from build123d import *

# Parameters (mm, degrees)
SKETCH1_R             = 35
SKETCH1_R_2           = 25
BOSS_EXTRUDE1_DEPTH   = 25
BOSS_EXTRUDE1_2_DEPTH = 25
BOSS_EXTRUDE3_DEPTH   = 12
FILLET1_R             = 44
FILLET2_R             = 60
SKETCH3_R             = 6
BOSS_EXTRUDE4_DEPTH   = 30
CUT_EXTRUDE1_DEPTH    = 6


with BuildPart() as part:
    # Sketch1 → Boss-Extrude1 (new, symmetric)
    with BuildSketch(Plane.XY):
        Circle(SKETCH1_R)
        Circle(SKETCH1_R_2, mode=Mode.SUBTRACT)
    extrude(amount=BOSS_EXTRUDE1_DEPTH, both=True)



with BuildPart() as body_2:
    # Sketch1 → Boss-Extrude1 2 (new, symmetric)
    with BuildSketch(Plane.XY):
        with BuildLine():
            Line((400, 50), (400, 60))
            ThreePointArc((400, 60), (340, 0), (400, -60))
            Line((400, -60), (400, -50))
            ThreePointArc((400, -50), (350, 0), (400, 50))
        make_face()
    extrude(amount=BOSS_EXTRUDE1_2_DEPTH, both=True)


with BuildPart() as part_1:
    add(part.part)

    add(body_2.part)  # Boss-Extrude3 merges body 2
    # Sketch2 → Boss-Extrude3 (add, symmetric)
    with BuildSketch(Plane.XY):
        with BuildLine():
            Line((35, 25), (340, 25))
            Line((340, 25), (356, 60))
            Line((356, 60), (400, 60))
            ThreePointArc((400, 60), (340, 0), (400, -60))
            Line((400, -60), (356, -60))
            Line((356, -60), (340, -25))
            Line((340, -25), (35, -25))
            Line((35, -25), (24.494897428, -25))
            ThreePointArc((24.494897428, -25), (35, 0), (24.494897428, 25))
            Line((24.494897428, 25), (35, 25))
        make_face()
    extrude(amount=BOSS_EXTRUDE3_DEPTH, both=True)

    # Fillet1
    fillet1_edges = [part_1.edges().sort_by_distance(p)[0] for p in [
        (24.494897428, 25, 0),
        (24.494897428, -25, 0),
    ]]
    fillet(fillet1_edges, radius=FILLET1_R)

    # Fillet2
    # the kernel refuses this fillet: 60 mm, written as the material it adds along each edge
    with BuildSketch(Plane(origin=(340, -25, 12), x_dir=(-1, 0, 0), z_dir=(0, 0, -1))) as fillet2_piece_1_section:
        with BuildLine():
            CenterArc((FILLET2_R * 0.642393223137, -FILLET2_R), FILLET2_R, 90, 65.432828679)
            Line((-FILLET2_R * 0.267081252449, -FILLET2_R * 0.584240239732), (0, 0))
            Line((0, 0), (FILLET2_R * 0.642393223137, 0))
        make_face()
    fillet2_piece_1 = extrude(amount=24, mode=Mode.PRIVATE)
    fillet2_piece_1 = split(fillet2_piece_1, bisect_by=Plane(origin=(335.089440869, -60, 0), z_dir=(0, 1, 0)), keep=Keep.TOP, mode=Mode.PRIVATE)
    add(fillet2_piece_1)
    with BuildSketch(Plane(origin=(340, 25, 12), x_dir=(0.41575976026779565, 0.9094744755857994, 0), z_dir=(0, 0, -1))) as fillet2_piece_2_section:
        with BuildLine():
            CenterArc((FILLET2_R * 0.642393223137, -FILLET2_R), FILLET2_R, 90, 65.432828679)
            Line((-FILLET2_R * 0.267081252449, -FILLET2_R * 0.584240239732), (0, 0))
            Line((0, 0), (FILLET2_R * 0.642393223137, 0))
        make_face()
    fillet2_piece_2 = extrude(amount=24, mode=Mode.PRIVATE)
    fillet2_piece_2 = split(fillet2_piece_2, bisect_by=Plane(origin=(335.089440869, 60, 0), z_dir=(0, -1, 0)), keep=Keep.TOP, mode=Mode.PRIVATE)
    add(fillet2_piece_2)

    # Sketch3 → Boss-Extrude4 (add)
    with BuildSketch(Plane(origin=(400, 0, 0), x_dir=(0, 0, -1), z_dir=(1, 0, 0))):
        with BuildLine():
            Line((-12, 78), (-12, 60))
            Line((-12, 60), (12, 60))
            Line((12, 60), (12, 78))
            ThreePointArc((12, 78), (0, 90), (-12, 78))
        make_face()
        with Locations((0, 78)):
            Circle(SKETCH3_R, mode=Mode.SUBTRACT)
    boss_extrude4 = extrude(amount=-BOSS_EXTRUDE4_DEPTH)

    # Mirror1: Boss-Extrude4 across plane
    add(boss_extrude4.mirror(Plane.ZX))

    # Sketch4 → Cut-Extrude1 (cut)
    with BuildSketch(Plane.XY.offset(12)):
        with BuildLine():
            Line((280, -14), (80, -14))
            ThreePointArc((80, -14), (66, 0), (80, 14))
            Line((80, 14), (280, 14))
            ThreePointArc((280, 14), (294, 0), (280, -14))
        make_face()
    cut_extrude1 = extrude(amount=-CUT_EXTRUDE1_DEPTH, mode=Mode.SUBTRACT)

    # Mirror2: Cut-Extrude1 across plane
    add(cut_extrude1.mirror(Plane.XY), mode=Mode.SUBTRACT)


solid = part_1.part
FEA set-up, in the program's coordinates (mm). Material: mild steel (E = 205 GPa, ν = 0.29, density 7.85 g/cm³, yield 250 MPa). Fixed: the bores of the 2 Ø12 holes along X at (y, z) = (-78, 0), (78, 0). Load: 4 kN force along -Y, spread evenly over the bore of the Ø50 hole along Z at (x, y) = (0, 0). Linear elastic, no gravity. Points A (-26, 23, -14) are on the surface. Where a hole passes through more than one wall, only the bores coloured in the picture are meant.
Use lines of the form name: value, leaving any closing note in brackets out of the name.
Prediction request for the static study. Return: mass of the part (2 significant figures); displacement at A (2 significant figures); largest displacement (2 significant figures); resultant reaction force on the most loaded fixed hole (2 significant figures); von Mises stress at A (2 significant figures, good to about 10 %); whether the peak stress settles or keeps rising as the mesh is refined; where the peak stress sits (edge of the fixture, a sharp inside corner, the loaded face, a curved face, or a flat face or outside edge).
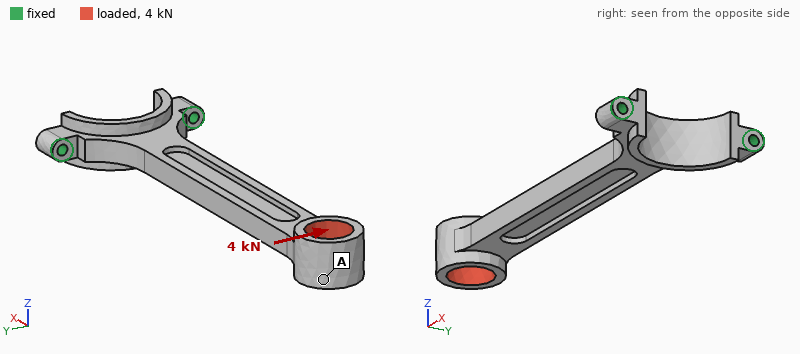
mass of the part: 4.3 kg
displacement at A: 1.5 mm
largest displacement: 1.5 mm
resultant reaction force on the most loaded fixed hole: 15 kN
von Mises stress at A: 12 MPa
whether the peak stress settles or keeps rising as the mesh is refined: keeps rising
where the peak stress sits: edge of the fixture
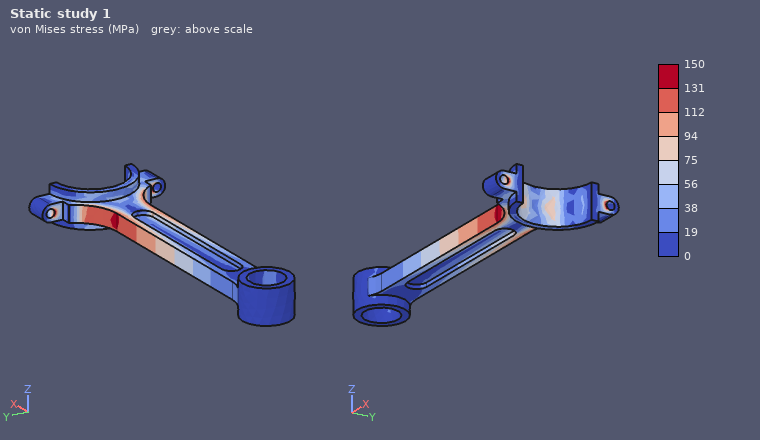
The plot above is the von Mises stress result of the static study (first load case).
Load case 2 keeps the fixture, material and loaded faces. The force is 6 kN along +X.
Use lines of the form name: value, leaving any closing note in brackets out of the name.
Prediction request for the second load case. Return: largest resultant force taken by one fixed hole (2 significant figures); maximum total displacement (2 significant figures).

largest resultant force taken by one fixed hole: 3.9 kN
maximum total displacement: 19 µm
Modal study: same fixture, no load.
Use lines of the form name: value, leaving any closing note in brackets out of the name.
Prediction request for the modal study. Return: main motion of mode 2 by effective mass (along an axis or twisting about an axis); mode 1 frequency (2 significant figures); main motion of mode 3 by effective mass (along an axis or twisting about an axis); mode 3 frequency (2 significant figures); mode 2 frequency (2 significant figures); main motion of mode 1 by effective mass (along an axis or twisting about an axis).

main motion of mode 2 by effective mass: along Y
mode 1 frequency: 94 Hz
main motion of mode 3 by effective mass: along Z
mode 3 frequency: 580 Hz
mode 2 frequency: 250 Hz
main motion of mode 1 by effective mass: along Z
